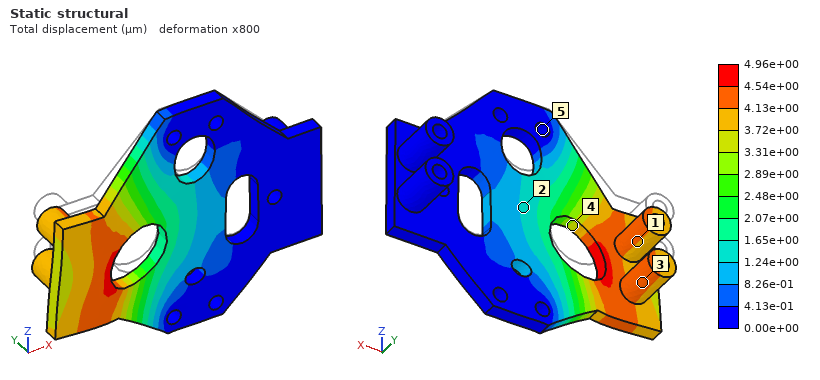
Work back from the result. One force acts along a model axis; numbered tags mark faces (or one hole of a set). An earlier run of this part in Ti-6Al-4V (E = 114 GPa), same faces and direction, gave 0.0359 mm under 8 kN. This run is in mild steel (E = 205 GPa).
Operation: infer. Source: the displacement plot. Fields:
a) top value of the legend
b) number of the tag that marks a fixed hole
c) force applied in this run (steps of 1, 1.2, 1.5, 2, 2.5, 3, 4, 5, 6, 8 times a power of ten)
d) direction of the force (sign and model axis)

4.96e+00 µm
5
2 kN
-Z
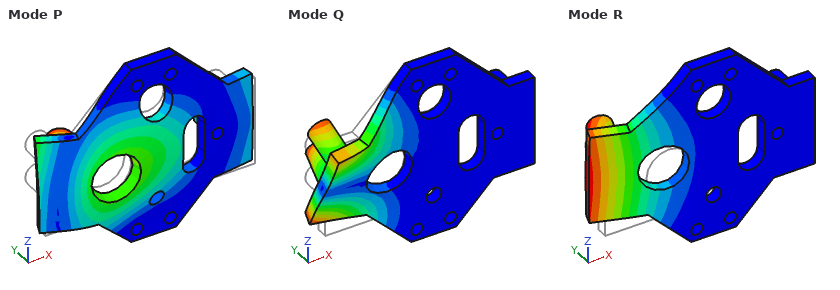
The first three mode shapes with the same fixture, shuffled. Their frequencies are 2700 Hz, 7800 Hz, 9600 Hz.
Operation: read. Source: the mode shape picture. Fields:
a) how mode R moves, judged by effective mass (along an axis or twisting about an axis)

along Y
